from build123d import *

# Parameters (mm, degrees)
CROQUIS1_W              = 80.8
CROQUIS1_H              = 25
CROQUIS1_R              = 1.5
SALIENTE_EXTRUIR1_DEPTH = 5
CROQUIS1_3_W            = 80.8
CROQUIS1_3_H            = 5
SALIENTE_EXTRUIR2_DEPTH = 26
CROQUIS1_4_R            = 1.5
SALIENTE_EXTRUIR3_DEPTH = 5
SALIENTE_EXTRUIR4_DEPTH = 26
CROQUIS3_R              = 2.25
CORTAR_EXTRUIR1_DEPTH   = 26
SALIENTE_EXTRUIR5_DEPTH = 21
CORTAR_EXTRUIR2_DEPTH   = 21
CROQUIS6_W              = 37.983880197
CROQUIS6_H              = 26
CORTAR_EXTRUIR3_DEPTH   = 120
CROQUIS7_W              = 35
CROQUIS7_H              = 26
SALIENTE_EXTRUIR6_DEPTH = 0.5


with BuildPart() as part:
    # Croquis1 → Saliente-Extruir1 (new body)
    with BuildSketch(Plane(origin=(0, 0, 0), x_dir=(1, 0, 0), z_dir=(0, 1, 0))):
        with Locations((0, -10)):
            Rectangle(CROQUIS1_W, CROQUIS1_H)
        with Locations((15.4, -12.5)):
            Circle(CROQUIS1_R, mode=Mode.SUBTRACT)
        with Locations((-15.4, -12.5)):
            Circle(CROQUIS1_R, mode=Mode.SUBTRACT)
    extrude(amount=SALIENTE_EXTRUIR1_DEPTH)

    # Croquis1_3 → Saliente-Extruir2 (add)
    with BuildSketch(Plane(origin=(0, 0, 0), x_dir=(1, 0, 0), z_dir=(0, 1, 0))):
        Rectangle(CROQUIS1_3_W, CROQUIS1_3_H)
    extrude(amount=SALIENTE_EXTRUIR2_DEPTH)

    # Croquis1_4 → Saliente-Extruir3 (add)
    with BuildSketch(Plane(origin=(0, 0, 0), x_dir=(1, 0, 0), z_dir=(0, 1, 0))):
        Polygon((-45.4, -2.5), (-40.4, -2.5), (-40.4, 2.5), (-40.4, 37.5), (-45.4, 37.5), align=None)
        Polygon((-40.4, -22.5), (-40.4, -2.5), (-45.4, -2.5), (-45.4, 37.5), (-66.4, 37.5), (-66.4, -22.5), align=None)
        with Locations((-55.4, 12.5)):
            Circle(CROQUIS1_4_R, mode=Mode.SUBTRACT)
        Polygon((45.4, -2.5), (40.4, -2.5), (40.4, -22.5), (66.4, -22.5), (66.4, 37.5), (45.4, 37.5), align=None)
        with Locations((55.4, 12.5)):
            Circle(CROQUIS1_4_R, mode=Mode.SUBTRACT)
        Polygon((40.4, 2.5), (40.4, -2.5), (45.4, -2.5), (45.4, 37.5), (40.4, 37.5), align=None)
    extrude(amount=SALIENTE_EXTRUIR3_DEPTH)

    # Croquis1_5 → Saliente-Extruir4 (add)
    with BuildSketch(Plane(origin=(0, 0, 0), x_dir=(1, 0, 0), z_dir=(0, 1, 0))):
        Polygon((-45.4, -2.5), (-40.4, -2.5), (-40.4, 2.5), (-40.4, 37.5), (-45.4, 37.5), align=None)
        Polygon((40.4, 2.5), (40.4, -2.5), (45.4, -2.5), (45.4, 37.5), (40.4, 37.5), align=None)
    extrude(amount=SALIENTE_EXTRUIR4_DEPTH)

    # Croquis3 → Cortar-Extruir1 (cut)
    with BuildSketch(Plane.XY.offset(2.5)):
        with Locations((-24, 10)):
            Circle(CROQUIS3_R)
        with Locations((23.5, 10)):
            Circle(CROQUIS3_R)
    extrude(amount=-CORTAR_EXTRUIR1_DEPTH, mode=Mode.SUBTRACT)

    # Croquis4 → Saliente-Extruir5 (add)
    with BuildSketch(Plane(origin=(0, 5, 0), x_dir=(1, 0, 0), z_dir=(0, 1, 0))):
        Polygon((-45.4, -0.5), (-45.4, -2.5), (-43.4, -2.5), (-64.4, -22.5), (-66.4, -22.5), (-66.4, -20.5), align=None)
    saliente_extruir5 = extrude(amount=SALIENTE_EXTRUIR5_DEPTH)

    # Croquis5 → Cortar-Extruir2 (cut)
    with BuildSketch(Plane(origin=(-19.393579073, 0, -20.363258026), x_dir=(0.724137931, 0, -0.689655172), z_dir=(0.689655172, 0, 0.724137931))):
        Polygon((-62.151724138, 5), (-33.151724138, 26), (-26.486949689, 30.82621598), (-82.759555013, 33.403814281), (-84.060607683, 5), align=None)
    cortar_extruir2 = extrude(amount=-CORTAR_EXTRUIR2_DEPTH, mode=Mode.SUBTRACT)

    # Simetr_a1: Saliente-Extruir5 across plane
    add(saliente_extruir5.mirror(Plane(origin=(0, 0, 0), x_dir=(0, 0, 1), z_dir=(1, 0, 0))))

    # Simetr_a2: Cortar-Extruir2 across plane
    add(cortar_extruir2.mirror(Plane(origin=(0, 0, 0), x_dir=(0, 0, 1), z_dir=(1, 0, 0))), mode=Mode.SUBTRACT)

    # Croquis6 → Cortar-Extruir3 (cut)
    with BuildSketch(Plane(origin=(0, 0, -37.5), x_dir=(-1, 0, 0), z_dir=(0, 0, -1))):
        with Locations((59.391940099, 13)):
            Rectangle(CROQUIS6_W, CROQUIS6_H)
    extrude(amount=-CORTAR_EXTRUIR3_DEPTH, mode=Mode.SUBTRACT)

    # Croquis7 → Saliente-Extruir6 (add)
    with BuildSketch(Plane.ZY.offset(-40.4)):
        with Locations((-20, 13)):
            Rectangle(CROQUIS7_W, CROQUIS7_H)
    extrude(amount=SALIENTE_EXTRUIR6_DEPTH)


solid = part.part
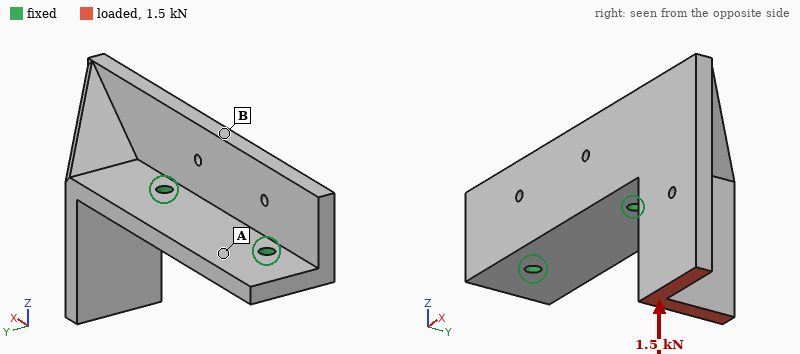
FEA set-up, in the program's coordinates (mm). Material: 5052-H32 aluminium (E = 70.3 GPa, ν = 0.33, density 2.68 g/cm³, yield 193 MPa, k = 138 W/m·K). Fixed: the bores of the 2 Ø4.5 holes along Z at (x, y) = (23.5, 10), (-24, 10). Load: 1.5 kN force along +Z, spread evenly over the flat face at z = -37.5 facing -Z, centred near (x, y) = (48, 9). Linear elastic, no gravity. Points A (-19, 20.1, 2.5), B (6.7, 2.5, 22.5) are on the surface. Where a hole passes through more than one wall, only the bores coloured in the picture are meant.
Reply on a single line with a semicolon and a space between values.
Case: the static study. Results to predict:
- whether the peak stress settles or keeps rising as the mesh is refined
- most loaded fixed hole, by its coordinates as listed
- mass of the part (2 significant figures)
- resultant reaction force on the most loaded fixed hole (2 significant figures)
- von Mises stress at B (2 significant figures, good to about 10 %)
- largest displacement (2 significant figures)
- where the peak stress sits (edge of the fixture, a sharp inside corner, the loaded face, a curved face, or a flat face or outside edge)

keeps rising; (23.5, 10); 85 g; 2.3 kN; 29 MPa; 0.14 mm; edge of the fixture
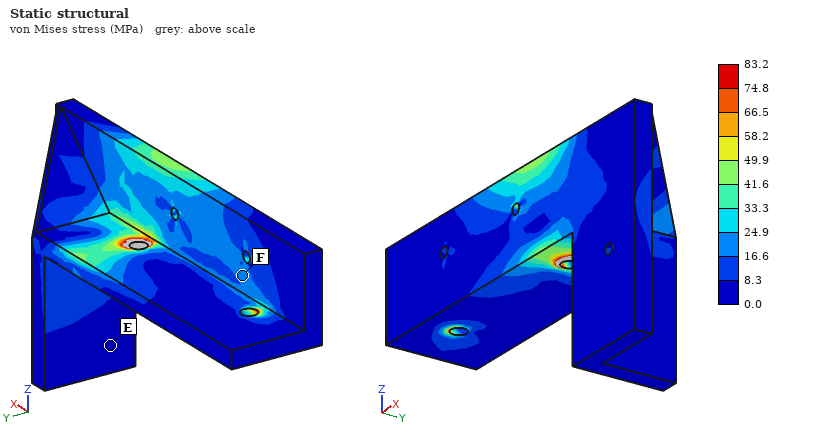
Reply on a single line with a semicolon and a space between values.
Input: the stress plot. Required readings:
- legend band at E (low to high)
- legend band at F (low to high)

0.0 to 8.3 MPa; 16.6 to 24.9 MPa
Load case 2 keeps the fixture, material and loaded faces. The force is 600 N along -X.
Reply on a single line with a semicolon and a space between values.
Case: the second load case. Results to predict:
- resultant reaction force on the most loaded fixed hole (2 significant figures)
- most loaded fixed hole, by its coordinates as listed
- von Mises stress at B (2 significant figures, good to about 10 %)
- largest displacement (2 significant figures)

1.2 kN; (23.5, 10); 19 MPa; 0.15 mm
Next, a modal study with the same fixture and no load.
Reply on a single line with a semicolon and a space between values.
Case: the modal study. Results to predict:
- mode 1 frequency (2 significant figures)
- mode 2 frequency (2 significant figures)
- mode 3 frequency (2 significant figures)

2000 Hz; 2800 Hz; 4200 Hz
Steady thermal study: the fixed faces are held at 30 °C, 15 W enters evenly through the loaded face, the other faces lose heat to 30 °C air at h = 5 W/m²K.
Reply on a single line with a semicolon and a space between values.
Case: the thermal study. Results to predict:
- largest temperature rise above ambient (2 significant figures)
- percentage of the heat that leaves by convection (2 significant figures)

30 K; 4.4 %
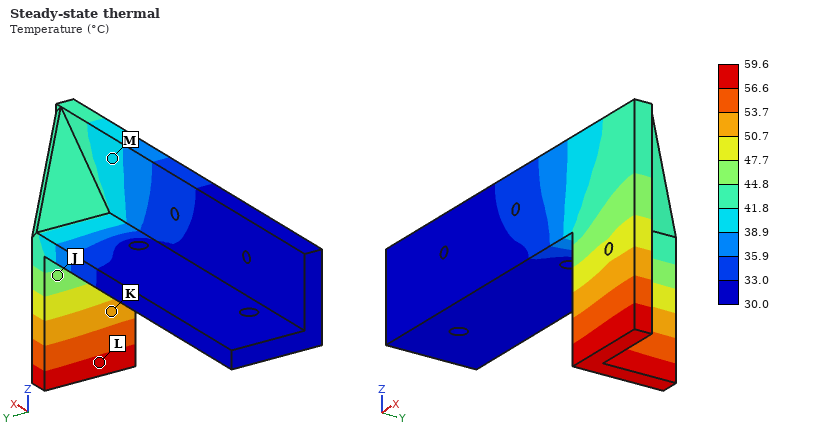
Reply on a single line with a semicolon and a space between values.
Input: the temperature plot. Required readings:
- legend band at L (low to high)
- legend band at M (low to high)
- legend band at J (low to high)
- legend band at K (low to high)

56.6 to 59.6 °C; 38.9 to 41.8 °C; 44.8 to 47.7 °C; 50.7 to 53.7 °C
